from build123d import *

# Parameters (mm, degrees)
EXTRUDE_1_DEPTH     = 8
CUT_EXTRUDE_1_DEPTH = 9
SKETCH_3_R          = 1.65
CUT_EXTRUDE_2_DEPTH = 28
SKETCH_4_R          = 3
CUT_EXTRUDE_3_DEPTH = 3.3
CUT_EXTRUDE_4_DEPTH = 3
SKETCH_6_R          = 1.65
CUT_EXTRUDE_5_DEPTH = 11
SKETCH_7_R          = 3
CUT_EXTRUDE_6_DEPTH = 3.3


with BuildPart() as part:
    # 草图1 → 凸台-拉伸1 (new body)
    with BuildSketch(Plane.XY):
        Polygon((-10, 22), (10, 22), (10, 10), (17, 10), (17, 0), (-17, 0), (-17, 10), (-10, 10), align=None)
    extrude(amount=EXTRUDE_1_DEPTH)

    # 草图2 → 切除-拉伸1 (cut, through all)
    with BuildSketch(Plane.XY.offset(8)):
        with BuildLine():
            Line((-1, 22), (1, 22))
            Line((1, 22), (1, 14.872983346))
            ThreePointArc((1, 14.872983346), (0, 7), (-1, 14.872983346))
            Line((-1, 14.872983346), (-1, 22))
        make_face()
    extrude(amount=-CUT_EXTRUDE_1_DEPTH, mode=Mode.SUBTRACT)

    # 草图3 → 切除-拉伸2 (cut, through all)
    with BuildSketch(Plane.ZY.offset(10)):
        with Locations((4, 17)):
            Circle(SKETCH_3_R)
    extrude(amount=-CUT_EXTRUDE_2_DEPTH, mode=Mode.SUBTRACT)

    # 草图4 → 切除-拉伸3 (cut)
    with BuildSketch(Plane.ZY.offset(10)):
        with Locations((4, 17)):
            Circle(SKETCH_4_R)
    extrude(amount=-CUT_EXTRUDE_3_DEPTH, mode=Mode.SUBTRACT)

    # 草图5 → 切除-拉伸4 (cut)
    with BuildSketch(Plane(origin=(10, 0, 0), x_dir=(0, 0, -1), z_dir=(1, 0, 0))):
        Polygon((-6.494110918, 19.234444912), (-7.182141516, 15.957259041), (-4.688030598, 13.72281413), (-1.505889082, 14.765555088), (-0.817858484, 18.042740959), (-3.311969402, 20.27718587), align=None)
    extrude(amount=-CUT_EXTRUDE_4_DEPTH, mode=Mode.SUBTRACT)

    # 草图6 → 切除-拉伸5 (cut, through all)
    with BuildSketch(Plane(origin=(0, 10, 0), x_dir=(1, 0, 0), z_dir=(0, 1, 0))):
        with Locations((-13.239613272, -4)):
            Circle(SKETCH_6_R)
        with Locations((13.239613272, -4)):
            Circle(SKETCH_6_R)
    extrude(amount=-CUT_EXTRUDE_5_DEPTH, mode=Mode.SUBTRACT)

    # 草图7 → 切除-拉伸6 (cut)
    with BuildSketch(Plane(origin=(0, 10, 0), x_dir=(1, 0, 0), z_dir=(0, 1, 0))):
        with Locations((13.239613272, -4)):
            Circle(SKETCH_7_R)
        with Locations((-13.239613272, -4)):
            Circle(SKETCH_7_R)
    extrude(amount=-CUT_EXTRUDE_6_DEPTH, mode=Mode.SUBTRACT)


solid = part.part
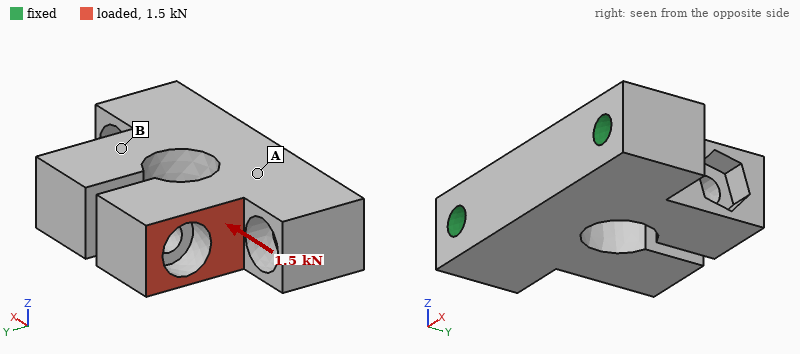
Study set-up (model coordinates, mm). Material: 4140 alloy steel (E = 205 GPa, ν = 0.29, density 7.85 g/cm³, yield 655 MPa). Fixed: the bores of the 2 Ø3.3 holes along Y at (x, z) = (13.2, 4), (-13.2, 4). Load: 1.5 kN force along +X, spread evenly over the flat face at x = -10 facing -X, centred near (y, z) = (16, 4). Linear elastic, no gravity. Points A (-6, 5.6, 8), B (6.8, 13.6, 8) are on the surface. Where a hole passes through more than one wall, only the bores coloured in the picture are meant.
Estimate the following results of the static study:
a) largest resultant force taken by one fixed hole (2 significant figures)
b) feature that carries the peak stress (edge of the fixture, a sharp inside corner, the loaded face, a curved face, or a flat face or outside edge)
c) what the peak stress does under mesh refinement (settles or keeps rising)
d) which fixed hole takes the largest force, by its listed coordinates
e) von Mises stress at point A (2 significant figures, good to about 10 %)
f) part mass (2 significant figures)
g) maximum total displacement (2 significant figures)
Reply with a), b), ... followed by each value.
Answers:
a) 1.2 kN
b) a sharp inside corner
c) keeps rising
d) (-13.2, 4)
e) 55 MPa
f) 28 g
g) 38 µm
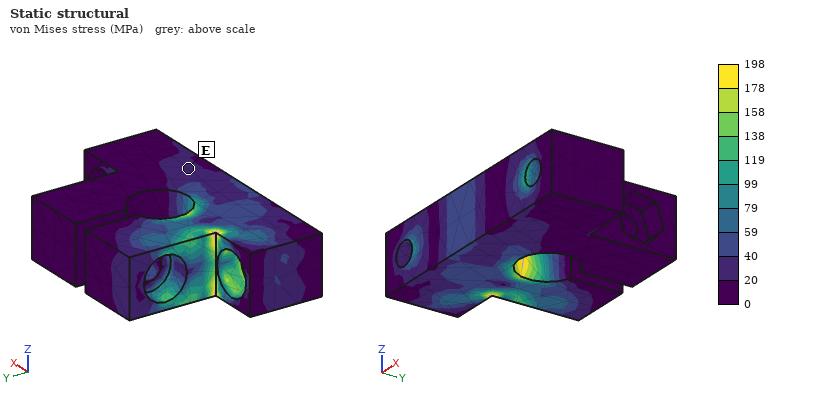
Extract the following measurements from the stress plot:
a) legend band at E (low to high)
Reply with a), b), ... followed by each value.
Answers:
a) 20 to 40 MPa
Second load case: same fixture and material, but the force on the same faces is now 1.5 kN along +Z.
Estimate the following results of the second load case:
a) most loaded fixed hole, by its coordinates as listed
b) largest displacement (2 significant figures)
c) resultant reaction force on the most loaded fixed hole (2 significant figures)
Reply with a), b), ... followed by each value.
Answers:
a) (-13.2, 4)
b) 63 µm
c) 1.4 kN
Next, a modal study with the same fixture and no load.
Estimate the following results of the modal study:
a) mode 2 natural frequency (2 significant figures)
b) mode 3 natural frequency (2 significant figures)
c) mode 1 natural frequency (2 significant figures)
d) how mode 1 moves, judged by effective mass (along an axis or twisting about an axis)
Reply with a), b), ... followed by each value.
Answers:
a) 14 kHz
b) 15 kHz
c) 12 kHz
d) along Z
